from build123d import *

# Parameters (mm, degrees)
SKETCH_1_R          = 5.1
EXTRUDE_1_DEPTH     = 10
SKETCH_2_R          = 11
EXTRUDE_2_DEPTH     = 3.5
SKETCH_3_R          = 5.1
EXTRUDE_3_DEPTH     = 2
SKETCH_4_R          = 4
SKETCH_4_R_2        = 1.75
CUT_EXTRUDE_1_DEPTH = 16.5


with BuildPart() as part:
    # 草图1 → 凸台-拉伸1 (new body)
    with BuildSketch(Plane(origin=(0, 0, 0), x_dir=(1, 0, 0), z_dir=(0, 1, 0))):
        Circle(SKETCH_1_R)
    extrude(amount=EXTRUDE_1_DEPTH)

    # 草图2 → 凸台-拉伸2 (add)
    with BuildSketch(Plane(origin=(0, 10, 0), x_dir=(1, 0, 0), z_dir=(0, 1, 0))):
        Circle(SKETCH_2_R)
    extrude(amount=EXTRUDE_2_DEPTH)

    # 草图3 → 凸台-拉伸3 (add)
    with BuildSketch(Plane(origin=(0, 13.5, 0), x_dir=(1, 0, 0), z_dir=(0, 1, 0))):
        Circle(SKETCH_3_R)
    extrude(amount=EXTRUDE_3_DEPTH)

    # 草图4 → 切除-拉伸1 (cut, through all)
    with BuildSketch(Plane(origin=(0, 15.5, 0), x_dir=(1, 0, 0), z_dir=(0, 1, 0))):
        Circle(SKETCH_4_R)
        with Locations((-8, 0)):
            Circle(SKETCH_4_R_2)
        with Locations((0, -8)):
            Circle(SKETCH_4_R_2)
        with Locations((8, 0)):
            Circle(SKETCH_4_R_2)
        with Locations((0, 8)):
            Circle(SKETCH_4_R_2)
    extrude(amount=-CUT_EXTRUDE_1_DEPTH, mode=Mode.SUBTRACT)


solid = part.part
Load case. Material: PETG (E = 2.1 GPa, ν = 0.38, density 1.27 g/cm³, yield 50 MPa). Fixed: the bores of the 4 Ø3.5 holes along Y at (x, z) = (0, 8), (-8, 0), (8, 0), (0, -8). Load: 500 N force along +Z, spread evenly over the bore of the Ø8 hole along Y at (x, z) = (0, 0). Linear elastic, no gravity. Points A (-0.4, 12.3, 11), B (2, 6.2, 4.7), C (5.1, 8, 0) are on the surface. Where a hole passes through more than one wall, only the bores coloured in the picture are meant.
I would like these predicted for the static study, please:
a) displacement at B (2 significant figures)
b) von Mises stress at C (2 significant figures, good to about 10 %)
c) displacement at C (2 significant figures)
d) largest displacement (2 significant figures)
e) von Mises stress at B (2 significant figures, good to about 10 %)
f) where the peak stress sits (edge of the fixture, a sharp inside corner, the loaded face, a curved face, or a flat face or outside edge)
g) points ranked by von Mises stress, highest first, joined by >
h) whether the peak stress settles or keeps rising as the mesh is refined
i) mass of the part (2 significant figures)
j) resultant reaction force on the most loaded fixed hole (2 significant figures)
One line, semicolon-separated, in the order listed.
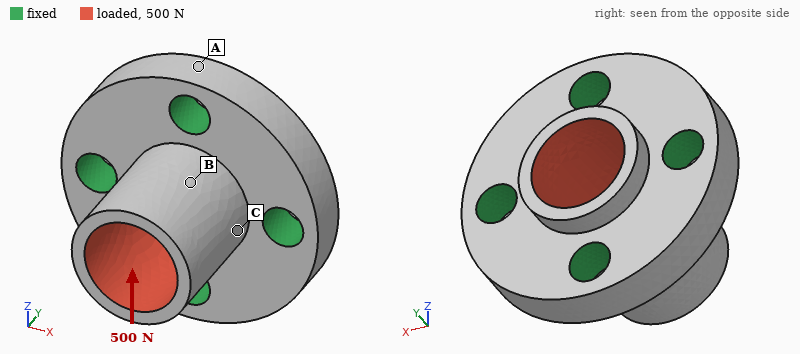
0.15 mm; 20 MPa; 0.072 mm; 0.28 mm; 11 MPa; a sharp inside corner; C > B > A; keeps rising; 1.8 g; 200 N
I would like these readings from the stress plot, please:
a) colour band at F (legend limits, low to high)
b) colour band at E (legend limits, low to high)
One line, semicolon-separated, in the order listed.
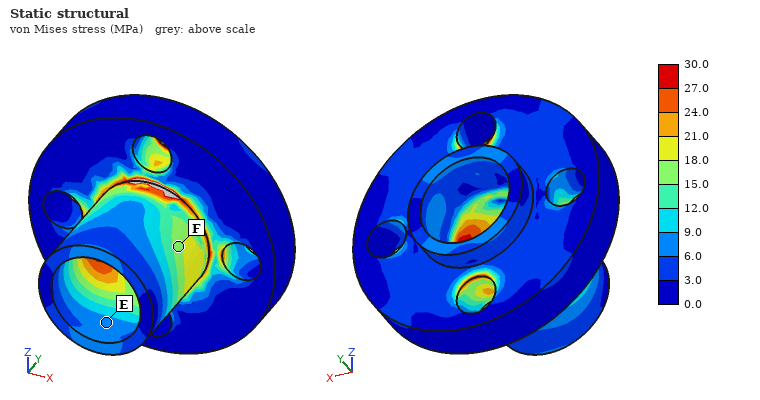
15.0 to 18.0 MPa; 6.0 to 9.0 MPa
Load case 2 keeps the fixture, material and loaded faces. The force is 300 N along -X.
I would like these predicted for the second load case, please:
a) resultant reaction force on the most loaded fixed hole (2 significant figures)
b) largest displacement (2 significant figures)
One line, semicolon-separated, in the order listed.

120 N; 0.17 mm
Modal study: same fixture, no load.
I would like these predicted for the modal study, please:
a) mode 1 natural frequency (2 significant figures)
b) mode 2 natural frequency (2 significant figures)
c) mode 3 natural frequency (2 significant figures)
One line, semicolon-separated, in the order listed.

10 kHz; 10 kHz; 11 kHz
